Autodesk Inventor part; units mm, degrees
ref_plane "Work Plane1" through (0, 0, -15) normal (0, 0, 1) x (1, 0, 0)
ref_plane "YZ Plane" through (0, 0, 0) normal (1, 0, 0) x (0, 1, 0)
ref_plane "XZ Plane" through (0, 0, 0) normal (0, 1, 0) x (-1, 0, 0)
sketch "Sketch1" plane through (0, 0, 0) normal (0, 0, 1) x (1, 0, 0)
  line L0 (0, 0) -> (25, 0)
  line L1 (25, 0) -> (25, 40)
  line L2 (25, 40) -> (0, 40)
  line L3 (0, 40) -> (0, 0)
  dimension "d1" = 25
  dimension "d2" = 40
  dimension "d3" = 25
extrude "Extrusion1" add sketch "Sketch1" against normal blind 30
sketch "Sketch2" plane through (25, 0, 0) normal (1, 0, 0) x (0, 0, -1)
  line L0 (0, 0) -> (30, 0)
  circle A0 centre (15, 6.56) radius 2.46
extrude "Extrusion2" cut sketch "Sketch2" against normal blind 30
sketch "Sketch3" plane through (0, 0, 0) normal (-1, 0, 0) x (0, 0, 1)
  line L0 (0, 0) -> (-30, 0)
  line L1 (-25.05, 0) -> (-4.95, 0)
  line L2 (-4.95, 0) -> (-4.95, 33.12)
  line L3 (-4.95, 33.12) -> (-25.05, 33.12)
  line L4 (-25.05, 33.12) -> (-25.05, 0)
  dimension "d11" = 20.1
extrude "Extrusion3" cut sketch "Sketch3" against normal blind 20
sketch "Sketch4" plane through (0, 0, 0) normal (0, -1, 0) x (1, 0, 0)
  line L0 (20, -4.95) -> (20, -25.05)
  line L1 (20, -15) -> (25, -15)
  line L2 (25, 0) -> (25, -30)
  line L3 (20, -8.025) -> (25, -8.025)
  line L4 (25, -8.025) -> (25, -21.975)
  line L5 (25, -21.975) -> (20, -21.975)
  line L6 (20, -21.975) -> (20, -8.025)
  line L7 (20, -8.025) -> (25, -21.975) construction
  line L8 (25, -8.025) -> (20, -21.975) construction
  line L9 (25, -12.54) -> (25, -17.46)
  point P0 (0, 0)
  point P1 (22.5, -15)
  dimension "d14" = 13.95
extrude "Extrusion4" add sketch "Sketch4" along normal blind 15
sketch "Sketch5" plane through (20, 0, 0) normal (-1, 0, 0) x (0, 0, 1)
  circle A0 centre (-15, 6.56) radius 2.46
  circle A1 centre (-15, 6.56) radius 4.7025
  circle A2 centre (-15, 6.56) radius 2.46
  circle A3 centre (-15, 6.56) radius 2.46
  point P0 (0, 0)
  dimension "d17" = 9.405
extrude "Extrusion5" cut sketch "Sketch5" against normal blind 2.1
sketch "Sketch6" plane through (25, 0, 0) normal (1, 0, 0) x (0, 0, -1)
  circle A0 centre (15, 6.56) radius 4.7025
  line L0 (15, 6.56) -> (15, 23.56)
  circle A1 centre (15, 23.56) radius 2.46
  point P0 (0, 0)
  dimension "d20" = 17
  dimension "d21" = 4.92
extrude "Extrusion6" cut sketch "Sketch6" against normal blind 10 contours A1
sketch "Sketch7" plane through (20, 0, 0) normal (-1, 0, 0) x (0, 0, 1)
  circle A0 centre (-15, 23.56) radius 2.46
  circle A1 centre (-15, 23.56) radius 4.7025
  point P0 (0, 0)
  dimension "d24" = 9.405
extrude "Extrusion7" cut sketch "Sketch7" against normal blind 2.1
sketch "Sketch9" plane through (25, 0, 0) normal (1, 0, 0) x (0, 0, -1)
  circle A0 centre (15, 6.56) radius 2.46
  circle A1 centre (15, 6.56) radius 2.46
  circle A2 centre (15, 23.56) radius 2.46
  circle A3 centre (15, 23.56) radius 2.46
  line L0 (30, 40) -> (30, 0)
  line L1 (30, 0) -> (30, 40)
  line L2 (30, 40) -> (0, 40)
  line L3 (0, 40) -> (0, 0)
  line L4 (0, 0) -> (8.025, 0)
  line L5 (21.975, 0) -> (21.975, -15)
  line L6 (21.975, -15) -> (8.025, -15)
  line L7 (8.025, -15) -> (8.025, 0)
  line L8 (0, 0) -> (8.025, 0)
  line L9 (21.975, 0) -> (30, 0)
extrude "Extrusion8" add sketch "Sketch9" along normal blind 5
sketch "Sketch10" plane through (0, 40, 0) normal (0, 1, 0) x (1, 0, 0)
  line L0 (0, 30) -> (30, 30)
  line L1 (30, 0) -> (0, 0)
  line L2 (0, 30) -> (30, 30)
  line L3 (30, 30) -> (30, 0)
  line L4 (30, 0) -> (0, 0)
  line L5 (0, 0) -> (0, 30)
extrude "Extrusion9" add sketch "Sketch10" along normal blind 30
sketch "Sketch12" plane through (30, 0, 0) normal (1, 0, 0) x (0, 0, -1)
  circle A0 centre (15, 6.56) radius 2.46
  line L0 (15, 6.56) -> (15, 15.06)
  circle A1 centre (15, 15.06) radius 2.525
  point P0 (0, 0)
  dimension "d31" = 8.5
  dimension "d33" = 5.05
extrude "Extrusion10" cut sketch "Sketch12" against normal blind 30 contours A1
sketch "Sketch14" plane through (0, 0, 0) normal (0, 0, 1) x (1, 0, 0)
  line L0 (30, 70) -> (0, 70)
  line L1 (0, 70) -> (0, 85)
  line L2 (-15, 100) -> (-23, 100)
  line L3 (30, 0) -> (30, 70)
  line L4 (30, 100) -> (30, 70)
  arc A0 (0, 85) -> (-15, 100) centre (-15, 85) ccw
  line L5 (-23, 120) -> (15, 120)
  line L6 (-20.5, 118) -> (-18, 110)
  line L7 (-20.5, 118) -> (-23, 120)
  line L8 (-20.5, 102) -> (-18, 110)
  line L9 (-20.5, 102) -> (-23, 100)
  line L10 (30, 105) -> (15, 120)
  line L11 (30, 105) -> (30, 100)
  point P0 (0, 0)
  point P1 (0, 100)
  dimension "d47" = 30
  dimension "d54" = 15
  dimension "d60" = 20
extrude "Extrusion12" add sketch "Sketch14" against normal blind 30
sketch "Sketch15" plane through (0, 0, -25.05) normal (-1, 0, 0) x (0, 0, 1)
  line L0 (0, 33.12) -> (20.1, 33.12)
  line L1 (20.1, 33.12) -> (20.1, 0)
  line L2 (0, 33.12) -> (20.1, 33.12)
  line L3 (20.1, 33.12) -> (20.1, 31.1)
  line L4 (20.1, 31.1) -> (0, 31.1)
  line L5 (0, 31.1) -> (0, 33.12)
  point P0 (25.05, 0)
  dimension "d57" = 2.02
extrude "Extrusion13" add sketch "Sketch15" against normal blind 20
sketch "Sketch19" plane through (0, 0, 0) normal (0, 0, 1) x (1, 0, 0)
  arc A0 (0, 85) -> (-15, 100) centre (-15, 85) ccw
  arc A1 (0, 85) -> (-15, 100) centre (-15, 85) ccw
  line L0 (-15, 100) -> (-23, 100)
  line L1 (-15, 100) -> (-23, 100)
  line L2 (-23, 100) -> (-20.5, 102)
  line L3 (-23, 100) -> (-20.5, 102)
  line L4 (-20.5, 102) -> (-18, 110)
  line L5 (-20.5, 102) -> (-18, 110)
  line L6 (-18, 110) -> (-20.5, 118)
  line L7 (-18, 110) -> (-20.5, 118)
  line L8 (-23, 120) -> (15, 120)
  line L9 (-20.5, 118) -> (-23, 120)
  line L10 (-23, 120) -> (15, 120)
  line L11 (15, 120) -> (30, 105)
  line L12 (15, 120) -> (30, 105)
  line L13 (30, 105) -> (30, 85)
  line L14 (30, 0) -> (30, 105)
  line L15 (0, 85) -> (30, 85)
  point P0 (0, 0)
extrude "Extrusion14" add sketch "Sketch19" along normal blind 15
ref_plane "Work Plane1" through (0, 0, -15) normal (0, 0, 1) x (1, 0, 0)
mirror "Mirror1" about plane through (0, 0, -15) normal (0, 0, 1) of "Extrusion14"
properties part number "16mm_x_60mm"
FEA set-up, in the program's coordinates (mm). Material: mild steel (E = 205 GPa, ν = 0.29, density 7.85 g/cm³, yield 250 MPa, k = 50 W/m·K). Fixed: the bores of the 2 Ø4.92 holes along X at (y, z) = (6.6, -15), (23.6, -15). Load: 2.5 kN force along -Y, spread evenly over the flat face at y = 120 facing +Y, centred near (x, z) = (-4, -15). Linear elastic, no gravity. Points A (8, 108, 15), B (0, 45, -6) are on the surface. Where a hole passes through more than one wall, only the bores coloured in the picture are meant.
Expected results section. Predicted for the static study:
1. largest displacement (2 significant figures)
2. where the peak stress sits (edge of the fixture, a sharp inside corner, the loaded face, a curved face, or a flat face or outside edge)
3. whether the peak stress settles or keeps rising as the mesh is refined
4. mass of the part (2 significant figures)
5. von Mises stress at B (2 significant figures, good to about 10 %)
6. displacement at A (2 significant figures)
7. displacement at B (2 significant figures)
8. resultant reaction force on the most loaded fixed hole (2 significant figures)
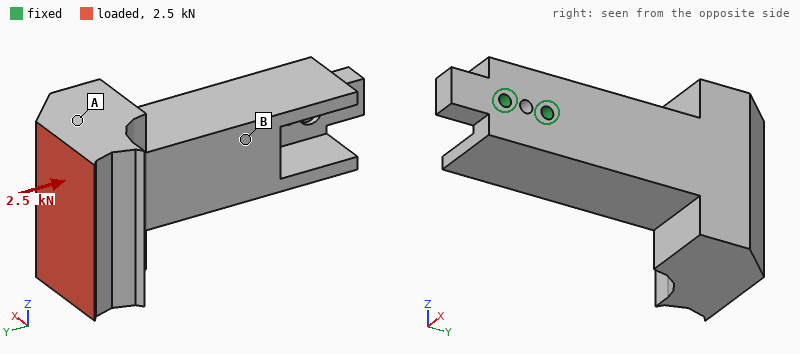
75 µm
edge of the fixture
keeps rising
1.2 kg
16 MPa
56 µm
19 µm
3.4 kN
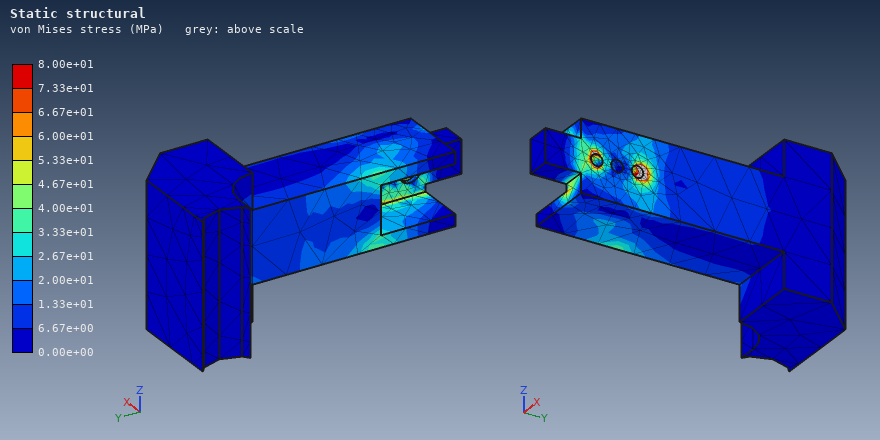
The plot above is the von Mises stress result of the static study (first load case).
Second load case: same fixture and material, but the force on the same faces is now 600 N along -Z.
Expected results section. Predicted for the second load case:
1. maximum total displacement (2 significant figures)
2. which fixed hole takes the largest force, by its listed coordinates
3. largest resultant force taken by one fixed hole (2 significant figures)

51 µm
(23.6, -15)
3.1 kN
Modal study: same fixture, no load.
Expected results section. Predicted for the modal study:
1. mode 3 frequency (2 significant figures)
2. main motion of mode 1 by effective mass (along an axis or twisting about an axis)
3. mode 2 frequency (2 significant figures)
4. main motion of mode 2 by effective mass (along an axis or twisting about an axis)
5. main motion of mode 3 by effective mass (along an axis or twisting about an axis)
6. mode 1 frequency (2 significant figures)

1800 Hz
along X
850 Hz
along Z
twisting about Y
740 Hz
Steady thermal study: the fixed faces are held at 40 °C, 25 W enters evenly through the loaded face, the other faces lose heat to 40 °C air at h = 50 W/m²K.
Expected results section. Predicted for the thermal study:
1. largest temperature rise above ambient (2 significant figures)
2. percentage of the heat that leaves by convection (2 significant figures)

31 K
67 %
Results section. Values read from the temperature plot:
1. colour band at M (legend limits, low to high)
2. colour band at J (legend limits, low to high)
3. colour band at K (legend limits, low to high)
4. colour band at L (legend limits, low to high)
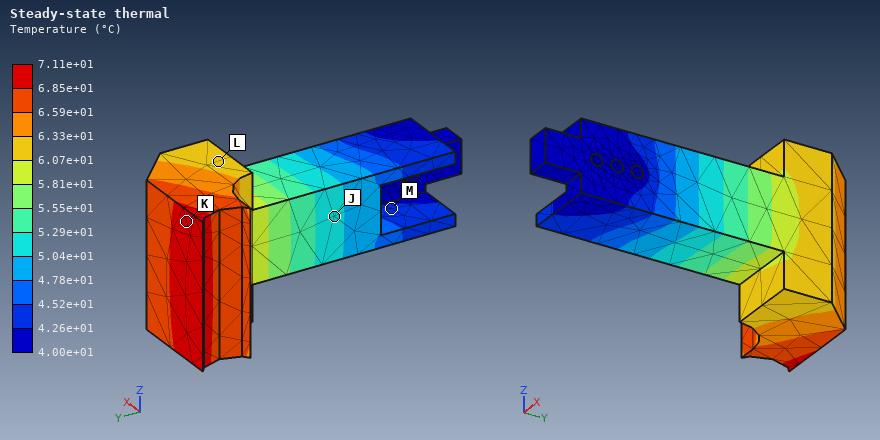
4.26e+01 to 4.52e+01 °C
5.04e+01 to 5.29e+01 °C
6.85e+01 to 7.11e+01 °C
6.07e+01 to 6.33e+01 °C
